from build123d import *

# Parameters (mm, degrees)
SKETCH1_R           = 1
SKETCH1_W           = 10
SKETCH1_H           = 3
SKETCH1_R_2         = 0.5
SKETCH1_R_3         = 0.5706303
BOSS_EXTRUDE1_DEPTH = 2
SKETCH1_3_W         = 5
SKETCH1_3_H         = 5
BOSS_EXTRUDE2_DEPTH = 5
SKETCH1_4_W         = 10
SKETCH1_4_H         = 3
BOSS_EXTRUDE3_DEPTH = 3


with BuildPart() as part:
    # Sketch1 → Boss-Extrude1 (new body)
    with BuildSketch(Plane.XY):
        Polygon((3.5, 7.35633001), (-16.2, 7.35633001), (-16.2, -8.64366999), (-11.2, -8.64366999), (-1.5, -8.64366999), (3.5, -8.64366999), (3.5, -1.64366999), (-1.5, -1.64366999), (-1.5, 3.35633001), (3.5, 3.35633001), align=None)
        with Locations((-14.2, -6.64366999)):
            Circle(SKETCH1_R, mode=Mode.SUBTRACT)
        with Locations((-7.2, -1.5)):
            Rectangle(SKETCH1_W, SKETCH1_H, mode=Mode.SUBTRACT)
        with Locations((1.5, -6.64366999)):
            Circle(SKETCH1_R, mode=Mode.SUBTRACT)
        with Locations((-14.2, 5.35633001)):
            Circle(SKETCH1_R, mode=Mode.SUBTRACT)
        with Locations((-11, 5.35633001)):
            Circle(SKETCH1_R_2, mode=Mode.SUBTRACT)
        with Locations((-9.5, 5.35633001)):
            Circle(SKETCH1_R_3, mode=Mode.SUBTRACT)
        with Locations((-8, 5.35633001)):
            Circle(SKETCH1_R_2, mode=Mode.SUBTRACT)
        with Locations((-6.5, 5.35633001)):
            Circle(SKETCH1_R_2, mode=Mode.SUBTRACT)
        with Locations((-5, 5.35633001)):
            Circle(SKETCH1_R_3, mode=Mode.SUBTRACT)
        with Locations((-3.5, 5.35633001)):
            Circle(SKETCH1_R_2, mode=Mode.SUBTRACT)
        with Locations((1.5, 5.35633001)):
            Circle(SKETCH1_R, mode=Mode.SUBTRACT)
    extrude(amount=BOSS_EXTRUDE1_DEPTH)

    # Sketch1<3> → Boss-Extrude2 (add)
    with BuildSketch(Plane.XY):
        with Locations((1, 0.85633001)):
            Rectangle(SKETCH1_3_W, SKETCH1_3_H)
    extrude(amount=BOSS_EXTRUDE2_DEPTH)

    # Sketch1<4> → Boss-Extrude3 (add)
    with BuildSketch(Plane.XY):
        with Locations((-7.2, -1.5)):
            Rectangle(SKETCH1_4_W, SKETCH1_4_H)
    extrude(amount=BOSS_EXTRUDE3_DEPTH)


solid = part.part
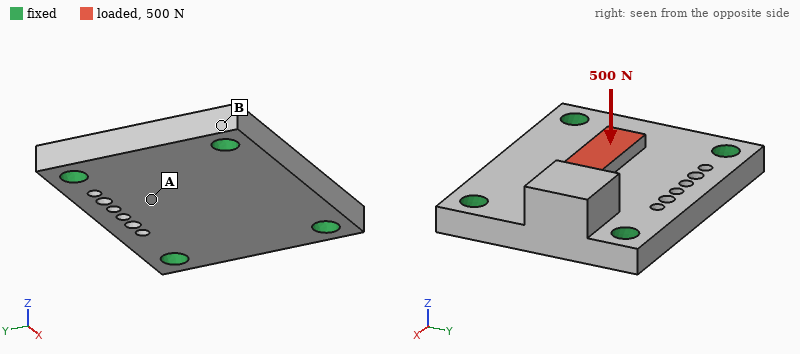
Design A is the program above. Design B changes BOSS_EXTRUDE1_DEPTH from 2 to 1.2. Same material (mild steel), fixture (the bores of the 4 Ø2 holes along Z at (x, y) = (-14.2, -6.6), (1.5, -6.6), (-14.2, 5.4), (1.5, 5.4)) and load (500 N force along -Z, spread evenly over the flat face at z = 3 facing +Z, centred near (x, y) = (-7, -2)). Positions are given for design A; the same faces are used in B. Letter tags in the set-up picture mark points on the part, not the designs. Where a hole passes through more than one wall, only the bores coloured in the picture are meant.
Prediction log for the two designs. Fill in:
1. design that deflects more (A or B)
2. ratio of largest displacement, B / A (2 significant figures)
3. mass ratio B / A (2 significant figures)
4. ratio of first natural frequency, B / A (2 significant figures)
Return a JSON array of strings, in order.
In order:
["B", "2.7", "0.72", "0.66"]
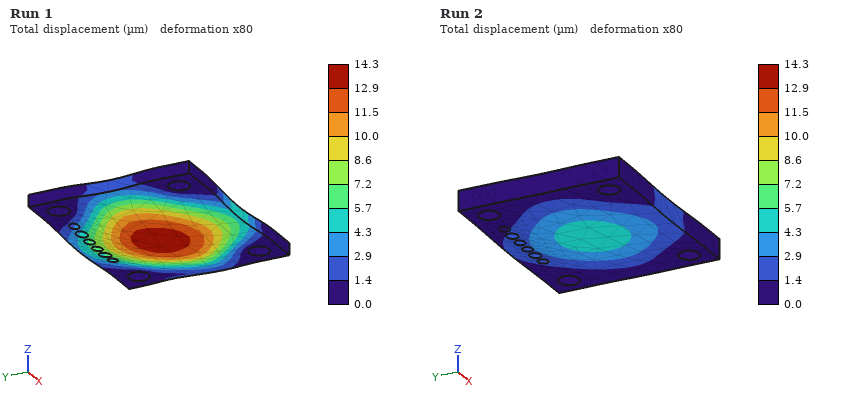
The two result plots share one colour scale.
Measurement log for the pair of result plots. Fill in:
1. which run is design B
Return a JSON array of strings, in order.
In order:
["Run 1"]
